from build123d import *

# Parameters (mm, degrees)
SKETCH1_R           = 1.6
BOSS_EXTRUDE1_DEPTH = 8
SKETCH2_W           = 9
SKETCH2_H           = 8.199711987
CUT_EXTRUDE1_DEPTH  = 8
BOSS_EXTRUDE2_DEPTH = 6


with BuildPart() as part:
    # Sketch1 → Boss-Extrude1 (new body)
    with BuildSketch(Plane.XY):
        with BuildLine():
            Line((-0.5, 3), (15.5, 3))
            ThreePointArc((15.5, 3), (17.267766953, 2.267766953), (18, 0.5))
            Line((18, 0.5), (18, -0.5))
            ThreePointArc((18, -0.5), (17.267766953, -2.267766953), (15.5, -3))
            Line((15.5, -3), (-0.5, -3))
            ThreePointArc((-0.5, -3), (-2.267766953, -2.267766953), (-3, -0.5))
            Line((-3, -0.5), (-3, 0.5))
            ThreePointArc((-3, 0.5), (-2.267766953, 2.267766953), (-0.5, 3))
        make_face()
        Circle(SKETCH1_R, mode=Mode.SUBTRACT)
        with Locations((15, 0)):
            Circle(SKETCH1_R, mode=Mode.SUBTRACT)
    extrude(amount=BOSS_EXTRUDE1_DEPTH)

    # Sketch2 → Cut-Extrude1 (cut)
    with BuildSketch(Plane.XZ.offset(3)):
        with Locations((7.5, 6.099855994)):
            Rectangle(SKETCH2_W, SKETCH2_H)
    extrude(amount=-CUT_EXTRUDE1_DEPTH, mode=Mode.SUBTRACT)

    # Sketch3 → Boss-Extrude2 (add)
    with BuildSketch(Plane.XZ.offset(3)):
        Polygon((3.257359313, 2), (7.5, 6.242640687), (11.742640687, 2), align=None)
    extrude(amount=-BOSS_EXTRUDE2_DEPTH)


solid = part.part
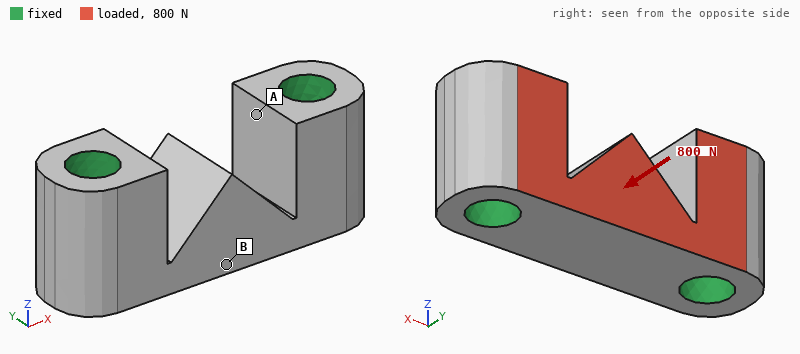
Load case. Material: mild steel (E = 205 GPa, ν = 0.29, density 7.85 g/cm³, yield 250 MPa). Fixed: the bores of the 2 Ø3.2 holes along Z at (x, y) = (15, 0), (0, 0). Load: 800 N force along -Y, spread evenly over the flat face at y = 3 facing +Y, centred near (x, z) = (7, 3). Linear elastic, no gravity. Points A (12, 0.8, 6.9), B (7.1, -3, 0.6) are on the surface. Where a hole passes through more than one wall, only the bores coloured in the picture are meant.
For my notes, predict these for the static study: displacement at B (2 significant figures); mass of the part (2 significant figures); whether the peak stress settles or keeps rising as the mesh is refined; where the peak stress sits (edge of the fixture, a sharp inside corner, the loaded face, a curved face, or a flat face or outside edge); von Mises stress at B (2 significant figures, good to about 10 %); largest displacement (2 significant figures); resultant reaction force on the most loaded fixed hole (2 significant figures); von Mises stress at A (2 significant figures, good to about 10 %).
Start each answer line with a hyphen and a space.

- 1.0 µm
- 4.9 g
- keeps rising
- a sharp inside corner
- 23 MPa
- 2.4 µm
- 400 N
- 6.7 MPa
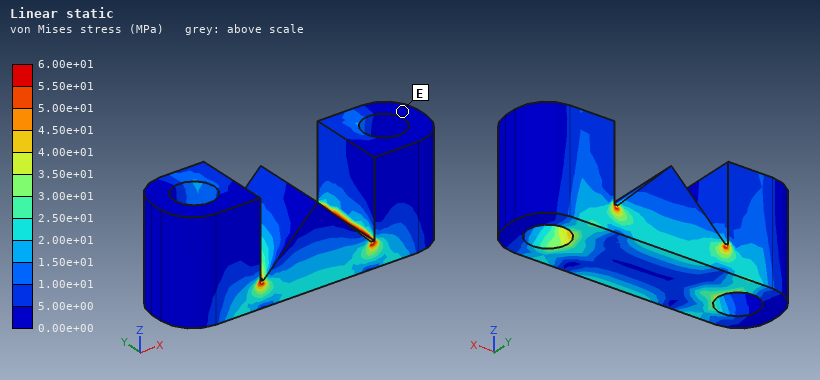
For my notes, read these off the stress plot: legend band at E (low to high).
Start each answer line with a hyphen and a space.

- 0.00e+00 to 5.00e+00 MPa
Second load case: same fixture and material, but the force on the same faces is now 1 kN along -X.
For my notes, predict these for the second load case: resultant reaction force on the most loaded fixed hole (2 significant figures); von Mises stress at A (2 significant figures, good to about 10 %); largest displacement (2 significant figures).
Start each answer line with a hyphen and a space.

- 510 N
- 14 MPa
- 1.2 µm
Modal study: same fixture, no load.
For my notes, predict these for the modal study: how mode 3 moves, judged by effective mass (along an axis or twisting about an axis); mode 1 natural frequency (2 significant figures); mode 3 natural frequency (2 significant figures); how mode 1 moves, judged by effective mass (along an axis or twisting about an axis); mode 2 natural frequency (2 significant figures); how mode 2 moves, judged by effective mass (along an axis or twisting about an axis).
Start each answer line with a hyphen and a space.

- along Y
- 55 kHz
- 95 kHz
- along Y
- 73 kHz
- along Z
